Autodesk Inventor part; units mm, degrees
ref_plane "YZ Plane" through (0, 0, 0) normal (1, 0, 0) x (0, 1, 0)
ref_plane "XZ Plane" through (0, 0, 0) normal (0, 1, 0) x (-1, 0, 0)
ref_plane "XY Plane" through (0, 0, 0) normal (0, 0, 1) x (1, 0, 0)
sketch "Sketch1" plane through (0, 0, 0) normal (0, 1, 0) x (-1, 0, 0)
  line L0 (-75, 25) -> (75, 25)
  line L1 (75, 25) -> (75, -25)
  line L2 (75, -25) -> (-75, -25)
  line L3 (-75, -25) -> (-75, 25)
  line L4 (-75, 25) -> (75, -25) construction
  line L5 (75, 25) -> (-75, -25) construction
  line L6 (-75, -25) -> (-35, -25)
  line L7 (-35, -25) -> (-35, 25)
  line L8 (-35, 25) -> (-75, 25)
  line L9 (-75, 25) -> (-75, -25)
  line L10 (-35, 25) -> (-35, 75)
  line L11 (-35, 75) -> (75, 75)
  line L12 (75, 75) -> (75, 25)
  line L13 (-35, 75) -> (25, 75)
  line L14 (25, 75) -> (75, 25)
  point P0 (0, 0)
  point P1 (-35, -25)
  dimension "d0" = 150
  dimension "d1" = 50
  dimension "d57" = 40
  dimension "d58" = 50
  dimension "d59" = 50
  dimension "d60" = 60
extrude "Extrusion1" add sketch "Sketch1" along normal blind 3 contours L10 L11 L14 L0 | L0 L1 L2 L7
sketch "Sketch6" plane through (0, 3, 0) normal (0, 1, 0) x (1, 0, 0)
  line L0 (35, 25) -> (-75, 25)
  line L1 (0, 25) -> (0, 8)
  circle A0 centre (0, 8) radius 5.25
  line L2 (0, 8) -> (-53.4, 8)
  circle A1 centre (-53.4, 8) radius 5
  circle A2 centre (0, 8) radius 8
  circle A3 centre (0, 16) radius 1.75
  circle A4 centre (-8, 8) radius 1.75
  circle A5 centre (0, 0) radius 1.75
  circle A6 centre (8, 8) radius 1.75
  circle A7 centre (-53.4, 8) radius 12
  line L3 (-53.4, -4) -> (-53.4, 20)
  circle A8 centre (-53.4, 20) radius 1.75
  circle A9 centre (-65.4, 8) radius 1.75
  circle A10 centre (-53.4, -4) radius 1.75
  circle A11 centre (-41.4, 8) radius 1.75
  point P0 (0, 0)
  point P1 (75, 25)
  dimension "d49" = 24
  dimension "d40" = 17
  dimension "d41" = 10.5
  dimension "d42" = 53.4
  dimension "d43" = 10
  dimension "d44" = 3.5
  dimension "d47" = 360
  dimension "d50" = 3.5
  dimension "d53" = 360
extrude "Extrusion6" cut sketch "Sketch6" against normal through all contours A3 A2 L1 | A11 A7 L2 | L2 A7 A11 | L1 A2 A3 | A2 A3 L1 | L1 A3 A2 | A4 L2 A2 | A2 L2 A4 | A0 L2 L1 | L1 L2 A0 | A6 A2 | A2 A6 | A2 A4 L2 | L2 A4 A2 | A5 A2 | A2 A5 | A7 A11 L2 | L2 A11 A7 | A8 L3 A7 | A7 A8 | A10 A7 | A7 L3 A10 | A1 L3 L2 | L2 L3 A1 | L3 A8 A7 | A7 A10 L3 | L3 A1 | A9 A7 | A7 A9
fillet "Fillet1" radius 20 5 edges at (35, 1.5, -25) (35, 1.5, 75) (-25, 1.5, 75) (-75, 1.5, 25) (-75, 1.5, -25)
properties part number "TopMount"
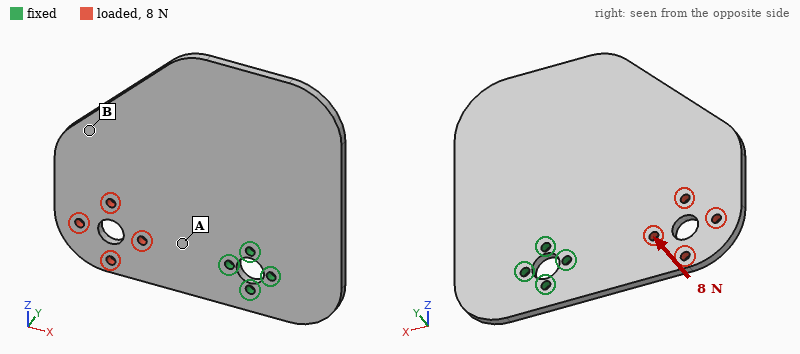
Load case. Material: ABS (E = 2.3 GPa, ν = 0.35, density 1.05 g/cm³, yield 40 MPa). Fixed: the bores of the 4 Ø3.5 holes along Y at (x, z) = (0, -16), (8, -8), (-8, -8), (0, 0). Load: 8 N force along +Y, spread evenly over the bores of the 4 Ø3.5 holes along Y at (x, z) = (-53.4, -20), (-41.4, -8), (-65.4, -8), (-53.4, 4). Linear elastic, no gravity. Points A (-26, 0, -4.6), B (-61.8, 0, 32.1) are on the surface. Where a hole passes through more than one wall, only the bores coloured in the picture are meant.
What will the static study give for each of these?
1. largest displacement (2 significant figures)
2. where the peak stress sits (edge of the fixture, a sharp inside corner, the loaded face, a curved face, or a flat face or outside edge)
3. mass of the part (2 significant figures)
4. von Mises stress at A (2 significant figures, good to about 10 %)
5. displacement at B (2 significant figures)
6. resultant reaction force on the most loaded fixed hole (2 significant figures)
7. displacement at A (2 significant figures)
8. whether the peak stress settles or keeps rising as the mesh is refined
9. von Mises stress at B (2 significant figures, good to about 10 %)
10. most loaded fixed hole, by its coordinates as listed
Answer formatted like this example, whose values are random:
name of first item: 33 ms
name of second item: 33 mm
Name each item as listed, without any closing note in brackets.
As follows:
largest displacement: 1.5 mm
where the peak stress sits: edge of the fixture
mass of the part: 29 g
von Mises stress at A: 2.2 MPa
displacement at B: 0.94 mm
resultant reaction force on the most loaded fixed hole: 23 N
displacement at A: 0.23 mm
whether the peak stress settles or keeps rising as the mesh is refined: keeps rising
von Mises stress at B: 0.70 MPa
most loaded fixed hole, by its coordinates as listed: (-8, -8)
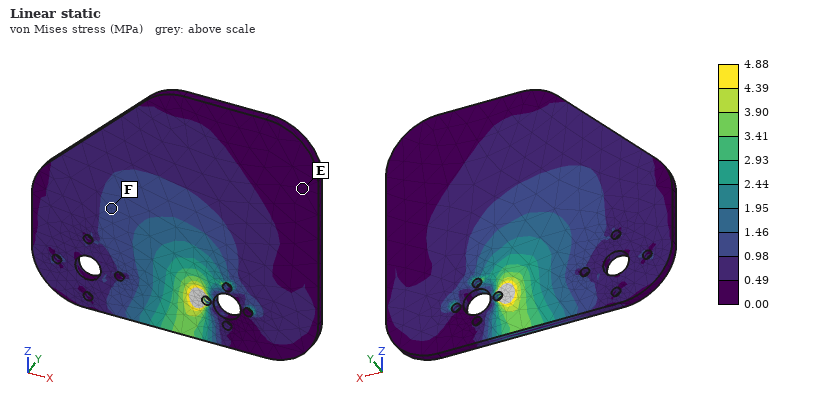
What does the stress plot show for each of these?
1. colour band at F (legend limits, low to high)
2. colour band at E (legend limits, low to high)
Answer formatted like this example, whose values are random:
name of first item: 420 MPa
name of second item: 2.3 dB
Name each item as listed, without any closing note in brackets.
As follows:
colour band at F: 0.98 to 1.46 MPa
colour band at E: 0.00 to 0.49 MPa
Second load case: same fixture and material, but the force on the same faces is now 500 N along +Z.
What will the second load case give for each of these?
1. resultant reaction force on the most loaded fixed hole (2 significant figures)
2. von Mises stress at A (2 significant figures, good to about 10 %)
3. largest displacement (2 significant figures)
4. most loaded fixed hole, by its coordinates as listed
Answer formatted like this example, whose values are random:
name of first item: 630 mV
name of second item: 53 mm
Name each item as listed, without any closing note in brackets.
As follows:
resultant reaction force on the most loaded fixed hole: 900 N
von Mises stress at A: 7.8 MPa
largest displacement: 1.2 mm
most loaded fixed hole, by its coordinates as listed: (-8, -8)
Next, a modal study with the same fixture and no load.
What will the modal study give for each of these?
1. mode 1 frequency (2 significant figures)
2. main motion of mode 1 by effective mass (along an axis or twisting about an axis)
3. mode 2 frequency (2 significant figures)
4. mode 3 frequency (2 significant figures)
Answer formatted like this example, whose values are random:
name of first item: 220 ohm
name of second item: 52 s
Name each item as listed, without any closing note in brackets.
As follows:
mode 1 frequency: 120 Hz
main motion of mode 1 by effective mass: along Y
mode 2 frequency: 150 Hz
mode 3 frequency: 310 Hz
